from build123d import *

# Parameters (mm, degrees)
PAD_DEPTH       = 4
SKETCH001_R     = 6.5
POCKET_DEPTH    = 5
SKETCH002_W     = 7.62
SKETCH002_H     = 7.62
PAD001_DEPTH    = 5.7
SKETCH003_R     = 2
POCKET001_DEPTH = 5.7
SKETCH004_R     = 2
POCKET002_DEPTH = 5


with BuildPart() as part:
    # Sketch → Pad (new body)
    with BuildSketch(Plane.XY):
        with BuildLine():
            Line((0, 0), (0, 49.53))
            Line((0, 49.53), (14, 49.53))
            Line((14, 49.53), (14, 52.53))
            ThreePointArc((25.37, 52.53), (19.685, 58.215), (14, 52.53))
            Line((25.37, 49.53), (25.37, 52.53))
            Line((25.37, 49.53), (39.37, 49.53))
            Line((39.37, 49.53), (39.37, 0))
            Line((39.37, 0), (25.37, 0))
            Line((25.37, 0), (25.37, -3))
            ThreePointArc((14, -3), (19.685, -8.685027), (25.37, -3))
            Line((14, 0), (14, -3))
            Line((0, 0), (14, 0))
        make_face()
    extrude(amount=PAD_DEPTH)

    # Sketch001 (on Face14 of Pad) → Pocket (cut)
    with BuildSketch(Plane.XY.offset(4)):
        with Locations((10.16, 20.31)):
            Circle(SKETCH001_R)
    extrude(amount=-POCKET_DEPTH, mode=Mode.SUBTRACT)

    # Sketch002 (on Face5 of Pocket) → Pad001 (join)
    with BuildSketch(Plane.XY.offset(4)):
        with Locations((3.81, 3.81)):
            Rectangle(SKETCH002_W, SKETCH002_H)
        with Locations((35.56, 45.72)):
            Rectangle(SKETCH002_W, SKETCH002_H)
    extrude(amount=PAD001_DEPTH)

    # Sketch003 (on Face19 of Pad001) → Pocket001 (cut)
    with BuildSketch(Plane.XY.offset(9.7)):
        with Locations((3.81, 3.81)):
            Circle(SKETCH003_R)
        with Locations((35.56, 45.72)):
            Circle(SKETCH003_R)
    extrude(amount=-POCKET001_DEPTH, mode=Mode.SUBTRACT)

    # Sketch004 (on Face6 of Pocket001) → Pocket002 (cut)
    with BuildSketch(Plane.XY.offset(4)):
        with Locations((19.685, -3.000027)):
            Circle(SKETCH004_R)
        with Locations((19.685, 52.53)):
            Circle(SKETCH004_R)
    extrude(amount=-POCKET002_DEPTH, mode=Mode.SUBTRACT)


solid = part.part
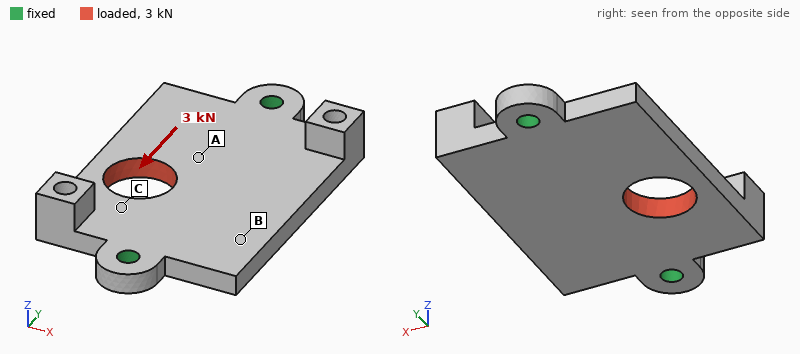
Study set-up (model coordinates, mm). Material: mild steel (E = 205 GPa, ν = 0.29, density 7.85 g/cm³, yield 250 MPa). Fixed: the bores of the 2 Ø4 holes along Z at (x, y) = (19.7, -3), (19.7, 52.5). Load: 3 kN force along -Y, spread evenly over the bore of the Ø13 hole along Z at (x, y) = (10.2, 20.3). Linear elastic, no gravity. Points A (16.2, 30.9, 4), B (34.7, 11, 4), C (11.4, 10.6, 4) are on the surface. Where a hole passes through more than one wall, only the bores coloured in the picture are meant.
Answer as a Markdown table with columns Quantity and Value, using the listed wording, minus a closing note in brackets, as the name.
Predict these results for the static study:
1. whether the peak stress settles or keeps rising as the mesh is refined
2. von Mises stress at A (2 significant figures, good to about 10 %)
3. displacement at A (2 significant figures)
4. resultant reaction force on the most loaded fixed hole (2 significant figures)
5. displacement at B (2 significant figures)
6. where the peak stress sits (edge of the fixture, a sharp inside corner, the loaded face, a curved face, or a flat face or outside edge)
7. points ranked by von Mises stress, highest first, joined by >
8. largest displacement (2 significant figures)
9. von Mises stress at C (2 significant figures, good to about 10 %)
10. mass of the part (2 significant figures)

| Quantity | Value |
|---|---|
| whether the peak stress settles or keeps rising as the mesh is refined | keeps rising |
| von Mises stress at A | 19 MPa |
| displacement at A | 2.4 µm |
| resultant reaction force on the most loaded fixed hole | 1.6 kN |
| displacement at B | 1.2 µm |
| where the peak stress sits | a sharp inside corner |
| points ranked by von Mises stress, highest first, joined by > | C > A > B |
| largest displacement | 6.1 µm |
| von Mises stress at C | 31 MPa |
| mass of the part | 66 g |
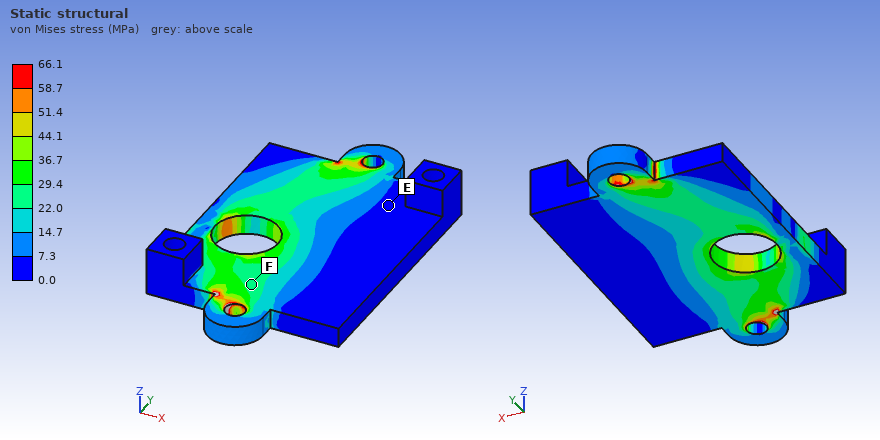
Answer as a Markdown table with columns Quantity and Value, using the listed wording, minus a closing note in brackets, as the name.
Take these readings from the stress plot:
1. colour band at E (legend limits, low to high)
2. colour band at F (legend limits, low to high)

| Quantity | Value |
|---|---|
| colour band at E | 0.0 to 7.3 MPa |
| colour band at F | 22.0 to 29.4 MPa |
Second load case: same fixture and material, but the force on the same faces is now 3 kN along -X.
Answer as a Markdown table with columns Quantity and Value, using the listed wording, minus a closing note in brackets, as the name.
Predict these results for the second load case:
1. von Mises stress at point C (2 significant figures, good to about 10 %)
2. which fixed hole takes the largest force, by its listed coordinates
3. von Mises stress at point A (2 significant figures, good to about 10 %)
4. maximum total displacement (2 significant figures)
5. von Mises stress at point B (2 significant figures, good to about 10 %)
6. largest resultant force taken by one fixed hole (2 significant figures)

| Quantity | Value |
|---|---|
| von Mises stress at point C | 32 MPa |
| which fixed hole takes the largest force, by its listed coordinates | (19.7, -3) |
| von Mises stress at point A | 17 MPa |
| maximum total displacement | 9.3 µm |
| von Mises stress at point B | 19 MPa |
| largest resultant force taken by one fixed hole | 1.8 kN |
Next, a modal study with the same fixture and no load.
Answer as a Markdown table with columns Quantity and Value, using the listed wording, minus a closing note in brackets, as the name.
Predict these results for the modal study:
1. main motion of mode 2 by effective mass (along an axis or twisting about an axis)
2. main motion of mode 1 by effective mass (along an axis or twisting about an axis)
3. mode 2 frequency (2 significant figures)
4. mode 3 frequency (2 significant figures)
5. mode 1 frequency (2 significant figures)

| Quantity | Value |
|---|---|
| main motion of mode 2 by effective mass | along Z |
| main motion of mode 1 by effective mass | twisting about Y |
| mode 2 frequency | 4600 Hz |
| mode 3 frequency | 7800 Hz |
| mode 1 frequency | 3700 Hz |
